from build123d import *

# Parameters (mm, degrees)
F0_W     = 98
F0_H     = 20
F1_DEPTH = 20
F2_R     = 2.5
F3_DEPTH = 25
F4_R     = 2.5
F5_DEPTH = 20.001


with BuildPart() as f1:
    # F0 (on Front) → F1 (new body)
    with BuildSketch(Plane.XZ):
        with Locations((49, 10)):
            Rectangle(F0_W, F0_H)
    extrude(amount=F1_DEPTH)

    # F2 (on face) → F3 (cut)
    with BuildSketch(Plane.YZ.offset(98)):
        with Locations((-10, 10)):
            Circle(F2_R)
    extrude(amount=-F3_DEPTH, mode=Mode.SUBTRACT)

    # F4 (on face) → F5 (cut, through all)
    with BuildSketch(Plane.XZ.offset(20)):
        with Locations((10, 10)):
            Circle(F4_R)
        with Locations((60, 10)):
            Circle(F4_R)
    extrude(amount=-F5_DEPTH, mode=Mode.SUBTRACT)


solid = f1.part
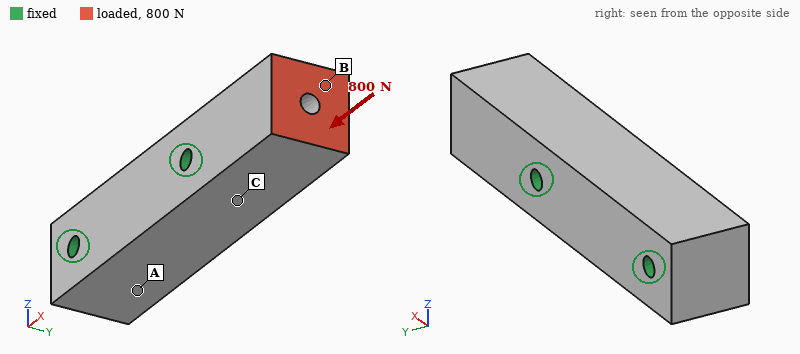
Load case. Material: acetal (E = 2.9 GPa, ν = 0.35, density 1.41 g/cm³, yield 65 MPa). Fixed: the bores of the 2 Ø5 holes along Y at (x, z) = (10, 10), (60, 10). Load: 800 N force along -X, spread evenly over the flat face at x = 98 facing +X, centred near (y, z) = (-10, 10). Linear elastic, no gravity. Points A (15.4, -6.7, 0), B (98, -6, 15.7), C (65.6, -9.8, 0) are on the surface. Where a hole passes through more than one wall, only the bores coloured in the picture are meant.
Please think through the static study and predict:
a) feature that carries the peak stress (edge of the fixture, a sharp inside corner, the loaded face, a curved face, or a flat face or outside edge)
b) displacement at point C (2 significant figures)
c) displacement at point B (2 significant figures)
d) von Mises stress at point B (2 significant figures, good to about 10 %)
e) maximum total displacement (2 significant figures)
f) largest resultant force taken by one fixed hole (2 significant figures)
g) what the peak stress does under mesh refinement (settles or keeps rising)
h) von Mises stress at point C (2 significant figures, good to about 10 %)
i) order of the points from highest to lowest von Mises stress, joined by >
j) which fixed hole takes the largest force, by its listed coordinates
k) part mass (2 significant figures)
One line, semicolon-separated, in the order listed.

edge of the fixture; 7.4 µm; 29 µm; 2.1 MPa; 29 µm; 750 N; keeps rising; 1.2 MPa; B > C > A; (60, 10); 53 g
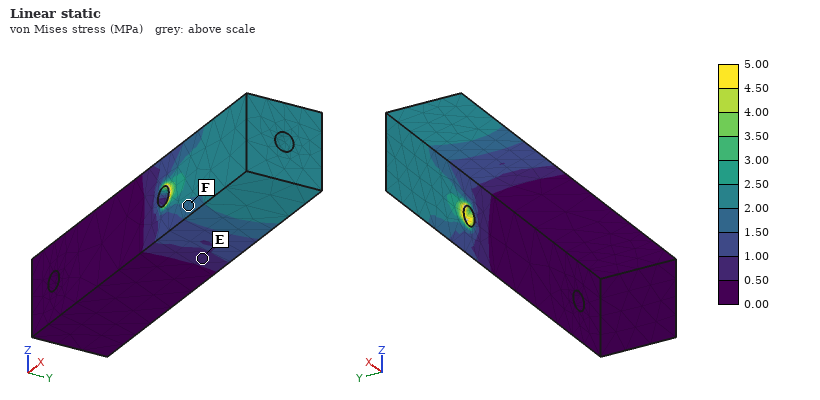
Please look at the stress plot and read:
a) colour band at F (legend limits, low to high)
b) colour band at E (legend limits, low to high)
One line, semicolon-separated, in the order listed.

1.50 to 2.00 MPa; 0.50 to 1.00 MPa
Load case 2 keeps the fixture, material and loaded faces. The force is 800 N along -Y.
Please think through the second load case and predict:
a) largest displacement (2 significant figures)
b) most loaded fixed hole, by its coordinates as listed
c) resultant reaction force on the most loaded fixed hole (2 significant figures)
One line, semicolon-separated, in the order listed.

0.54 mm; (60, 10); 910 N
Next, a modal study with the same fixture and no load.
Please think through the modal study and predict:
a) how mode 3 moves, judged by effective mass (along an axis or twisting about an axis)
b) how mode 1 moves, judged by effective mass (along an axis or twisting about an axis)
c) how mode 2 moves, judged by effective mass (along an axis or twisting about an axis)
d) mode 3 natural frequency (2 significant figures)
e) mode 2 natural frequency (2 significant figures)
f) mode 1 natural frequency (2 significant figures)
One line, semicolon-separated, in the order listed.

twisting about X; along Z; along Y; 5200 Hz; 2600 Hz; 2100 Hz
